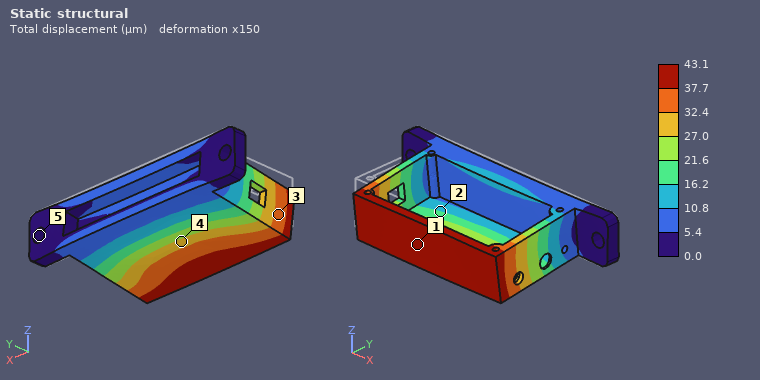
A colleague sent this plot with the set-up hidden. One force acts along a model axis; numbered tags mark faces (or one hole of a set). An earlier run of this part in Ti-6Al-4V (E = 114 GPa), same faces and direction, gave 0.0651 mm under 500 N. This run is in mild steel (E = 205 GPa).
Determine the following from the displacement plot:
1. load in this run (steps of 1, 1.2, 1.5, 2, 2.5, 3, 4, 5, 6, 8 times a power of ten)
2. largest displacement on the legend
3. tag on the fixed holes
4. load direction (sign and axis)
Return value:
600 N
43.1 µm
5
-Z
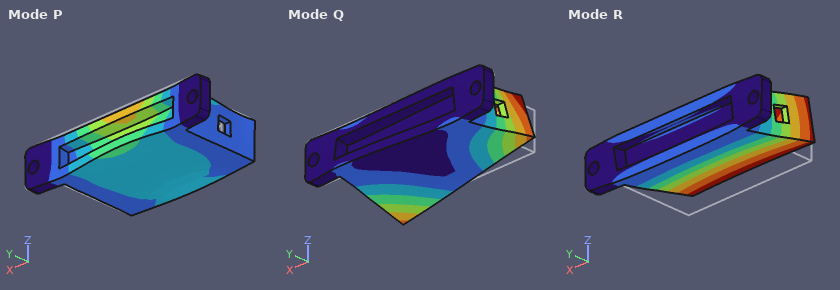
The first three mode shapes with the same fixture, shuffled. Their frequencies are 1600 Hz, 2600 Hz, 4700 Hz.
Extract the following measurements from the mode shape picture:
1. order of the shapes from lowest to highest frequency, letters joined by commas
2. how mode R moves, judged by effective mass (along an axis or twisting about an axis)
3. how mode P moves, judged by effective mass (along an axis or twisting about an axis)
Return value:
R, Q, P
along Z
along Y
